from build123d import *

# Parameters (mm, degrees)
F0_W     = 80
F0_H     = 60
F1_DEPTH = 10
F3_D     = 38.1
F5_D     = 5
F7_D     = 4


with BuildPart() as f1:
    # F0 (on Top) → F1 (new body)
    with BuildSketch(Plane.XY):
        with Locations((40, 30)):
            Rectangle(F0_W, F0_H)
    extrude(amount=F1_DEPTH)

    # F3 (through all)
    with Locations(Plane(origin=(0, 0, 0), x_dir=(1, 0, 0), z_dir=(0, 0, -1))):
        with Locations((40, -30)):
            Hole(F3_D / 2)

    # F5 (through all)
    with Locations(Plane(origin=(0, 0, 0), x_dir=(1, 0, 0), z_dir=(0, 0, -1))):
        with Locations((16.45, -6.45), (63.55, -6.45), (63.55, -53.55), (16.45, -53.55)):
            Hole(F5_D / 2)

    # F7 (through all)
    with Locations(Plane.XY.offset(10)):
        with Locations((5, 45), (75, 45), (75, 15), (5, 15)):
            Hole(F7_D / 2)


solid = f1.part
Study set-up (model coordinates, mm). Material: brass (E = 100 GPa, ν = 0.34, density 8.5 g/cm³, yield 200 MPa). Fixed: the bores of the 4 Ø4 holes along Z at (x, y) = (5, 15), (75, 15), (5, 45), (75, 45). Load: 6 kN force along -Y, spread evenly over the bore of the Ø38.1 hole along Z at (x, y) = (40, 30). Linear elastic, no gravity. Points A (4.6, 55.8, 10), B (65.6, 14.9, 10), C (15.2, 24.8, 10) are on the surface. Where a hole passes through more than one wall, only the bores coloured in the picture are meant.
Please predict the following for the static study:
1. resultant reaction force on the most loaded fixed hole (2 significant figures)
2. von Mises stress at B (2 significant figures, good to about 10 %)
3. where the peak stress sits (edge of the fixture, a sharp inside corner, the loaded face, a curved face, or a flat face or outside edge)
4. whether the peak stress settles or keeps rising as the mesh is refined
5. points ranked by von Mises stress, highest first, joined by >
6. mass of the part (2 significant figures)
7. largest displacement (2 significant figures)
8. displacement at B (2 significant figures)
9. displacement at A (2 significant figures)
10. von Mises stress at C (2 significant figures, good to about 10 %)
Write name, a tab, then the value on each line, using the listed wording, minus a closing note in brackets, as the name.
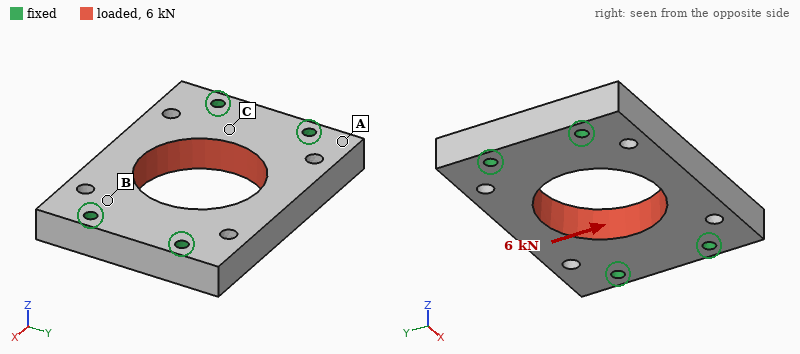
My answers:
resultant reaction force on the most loaded fixed hole	1.6 kN
von Mises stress at B	8.4 MPa
where the peak stress sits	edge of the fixture
whether the peak stress settles or keeps rising as the mesh is refined	keeps rising
points ranked by von Mises stress, highest first, joined by >	C > B > A
mass of the part	300 g
largest displacement	8.2 µm
displacement at B	2.3 µm
displacement at A	1.7 µm
von Mises stress at C	16 MPa
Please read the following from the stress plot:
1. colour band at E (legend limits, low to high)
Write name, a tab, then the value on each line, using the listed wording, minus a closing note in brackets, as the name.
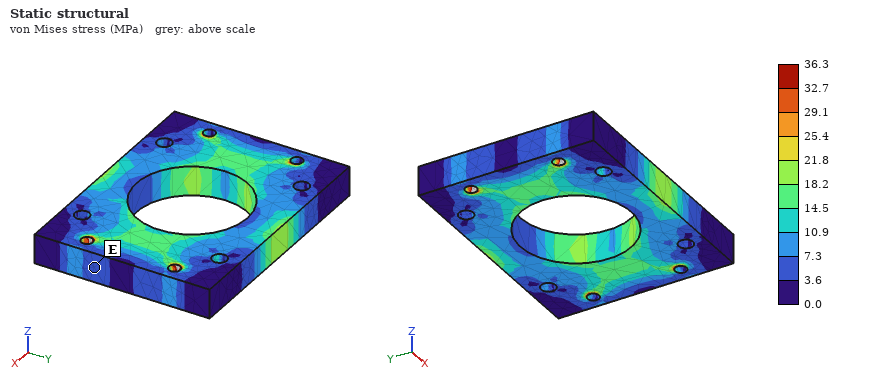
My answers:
colour band at E	3.6 to 7.3 MPa
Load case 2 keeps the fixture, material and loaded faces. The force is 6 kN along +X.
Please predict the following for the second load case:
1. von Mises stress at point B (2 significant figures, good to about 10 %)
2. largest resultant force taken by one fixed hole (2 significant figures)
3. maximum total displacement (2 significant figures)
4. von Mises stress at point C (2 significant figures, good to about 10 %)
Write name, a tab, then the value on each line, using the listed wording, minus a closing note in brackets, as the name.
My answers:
von Mises stress at point B	10 MPa
largest resultant force taken by one fixed hole	1.5 kN
maximum total displacement	2.9 µm
von Mises stress at point C	4.6 MPa
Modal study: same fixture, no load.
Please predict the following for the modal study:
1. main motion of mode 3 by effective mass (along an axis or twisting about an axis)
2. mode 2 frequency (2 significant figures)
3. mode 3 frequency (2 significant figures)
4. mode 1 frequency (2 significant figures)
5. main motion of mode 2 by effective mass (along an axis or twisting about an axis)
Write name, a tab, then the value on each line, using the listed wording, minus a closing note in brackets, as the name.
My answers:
main motion of mode 3 by effective mass	twisting about Y
mode 2 frequency	6300 Hz
mode 3 frequency	13 kHz
mode 1 frequency	6000 Hz
main motion of mode 2 by effective mass	twisting about X
